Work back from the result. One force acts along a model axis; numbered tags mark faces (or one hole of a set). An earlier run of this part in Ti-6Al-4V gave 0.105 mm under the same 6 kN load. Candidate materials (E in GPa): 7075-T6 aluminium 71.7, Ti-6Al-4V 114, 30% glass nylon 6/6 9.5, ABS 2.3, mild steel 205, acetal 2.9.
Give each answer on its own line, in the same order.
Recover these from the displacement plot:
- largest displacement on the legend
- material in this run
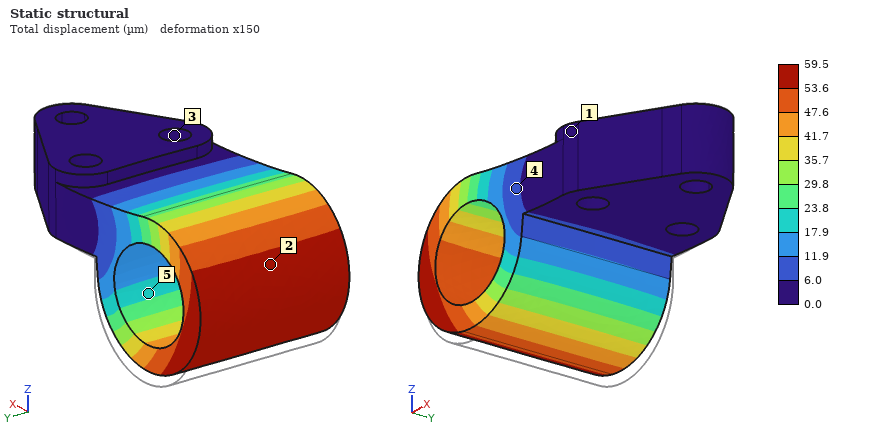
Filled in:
59.5 µm
mild steel
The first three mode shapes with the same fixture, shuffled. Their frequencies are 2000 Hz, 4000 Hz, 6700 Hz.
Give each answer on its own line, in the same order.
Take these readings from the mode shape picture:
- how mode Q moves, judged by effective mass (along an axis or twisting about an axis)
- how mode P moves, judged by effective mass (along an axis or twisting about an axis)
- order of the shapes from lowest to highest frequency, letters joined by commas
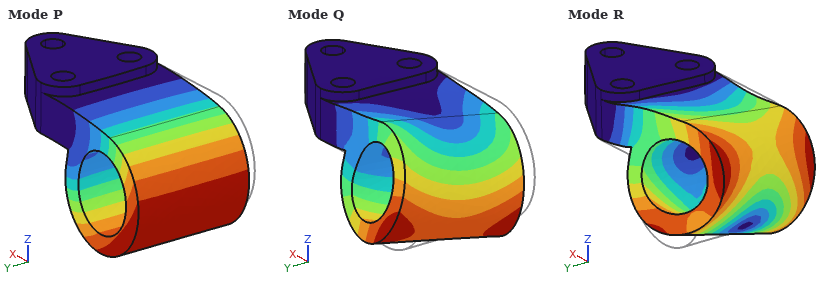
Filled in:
along Y
along Z
P, Q, R
